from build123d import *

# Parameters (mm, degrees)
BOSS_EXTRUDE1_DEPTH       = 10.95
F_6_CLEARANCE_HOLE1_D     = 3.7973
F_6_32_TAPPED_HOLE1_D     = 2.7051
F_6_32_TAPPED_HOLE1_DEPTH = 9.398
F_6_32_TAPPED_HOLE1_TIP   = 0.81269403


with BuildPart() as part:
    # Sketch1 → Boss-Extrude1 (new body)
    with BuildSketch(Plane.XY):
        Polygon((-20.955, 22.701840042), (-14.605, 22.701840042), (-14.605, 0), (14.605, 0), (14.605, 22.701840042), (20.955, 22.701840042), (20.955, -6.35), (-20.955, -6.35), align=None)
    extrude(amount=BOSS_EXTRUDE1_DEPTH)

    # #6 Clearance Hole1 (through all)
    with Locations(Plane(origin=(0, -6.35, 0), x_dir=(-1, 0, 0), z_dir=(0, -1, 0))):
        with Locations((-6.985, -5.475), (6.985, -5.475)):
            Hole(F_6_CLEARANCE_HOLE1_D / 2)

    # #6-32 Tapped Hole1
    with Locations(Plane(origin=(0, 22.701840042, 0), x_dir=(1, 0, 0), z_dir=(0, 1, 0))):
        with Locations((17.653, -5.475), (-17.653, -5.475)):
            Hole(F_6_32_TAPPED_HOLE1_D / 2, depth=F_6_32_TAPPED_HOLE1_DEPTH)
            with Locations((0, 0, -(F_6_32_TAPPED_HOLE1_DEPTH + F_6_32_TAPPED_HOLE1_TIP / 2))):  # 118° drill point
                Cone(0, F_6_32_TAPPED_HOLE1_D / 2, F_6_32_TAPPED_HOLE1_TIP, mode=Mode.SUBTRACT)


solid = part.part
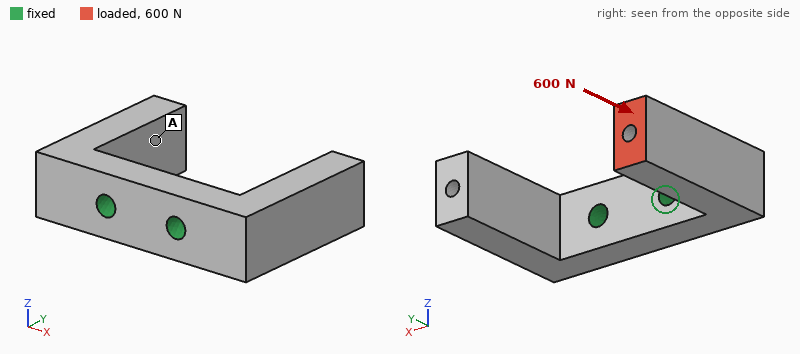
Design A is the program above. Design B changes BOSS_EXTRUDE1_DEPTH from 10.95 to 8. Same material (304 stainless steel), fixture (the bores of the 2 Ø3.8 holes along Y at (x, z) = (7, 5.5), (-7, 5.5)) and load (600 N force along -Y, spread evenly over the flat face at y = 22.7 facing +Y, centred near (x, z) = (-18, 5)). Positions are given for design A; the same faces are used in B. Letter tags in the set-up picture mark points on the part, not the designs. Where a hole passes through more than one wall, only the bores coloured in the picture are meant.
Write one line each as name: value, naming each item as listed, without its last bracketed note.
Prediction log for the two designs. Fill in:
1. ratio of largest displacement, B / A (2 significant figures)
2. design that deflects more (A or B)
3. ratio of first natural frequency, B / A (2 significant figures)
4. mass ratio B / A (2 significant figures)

ratio of largest displacement, B / A: 1.3
design that deflects more: B
ratio of first natural frequency, B / A: 1.0
mass ratio B / A: 0.72
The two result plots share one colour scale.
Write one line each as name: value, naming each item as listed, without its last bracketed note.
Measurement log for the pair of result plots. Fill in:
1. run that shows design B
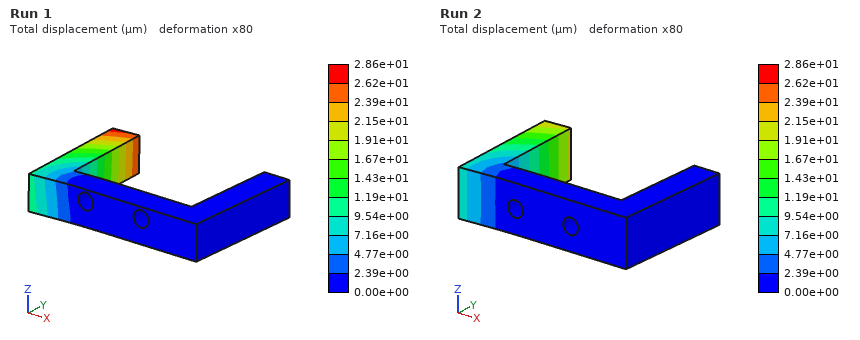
run that shows design B: Run 1
